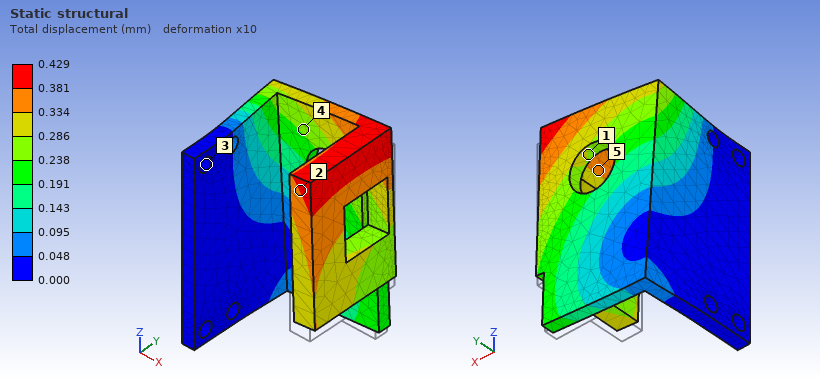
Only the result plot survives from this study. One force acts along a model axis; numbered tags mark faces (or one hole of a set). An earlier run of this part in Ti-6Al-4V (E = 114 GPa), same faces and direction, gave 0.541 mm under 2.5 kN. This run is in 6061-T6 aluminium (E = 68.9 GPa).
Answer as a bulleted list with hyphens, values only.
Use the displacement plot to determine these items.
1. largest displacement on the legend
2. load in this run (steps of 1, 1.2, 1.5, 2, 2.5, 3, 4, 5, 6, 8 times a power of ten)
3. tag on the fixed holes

- 0.429 mm
- 1.2 kN
- 3
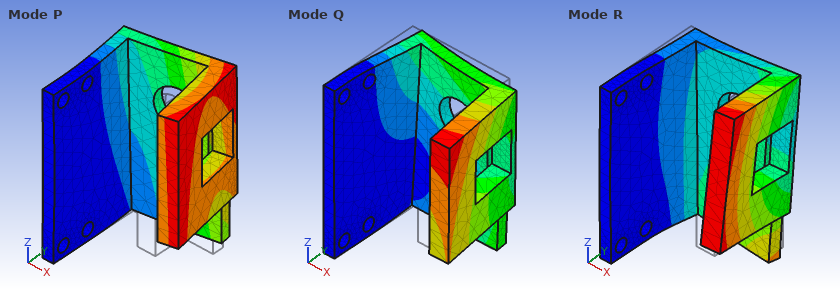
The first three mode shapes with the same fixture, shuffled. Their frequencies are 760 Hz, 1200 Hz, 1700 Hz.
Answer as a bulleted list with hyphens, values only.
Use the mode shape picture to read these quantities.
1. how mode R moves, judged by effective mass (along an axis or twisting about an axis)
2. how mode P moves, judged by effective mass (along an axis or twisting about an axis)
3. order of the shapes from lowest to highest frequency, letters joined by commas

- along X
- along Y
- P, Q, R
